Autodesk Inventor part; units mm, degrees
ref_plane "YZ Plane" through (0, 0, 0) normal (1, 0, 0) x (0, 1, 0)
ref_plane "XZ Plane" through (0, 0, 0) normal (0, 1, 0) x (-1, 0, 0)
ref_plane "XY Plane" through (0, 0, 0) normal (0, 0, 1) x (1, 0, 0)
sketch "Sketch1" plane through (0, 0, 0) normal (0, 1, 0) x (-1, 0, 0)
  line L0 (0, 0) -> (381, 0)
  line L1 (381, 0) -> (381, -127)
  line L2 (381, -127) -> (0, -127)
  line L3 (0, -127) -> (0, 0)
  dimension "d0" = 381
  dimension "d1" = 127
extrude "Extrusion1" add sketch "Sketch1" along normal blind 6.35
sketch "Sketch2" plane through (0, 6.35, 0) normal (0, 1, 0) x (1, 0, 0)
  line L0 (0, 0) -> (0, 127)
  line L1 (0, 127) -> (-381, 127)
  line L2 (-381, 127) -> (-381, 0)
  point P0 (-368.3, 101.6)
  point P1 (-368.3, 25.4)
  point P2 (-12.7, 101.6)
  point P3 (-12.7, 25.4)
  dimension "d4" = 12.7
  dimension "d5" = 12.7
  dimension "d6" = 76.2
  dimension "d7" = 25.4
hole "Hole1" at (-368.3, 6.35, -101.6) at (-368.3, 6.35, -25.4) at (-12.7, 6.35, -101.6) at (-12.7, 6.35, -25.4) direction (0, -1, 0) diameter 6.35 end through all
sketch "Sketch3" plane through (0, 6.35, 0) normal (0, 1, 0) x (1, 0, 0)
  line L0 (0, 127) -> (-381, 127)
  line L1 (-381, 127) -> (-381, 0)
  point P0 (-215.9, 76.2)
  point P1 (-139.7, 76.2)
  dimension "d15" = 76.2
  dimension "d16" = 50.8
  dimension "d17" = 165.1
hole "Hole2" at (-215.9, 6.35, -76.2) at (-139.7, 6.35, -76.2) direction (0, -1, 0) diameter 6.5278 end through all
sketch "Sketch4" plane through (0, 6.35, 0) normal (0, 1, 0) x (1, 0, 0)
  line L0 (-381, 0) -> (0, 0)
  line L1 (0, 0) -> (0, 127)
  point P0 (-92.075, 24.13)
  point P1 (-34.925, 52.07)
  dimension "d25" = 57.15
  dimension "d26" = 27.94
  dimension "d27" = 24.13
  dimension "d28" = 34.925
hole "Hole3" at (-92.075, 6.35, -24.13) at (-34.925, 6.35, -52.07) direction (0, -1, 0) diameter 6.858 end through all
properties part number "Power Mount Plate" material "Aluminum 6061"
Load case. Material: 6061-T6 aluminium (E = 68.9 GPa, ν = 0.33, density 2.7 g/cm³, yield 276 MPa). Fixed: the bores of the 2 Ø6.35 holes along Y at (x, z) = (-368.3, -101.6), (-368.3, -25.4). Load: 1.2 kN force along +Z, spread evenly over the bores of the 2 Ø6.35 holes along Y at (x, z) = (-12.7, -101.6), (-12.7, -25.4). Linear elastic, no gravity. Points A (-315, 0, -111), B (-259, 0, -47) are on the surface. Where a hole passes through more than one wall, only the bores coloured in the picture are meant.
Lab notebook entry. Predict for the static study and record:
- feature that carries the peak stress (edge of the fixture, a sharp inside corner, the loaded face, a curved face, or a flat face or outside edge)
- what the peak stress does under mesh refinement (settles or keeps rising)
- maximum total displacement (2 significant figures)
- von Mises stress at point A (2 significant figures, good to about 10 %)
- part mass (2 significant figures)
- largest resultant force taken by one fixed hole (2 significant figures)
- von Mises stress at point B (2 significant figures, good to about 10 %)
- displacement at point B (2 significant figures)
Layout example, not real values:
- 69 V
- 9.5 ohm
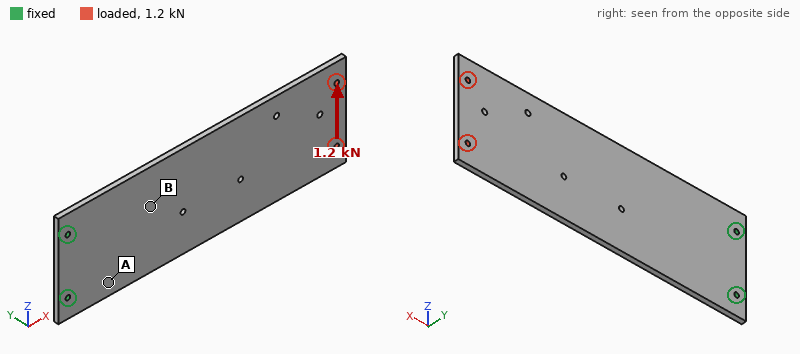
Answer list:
- edge of the fixture
- keeps rising
- 0.36 mm
- 16 MPa
- 830 g
- 5.4 kN
- 5.7 MPa
- 0.060 mm
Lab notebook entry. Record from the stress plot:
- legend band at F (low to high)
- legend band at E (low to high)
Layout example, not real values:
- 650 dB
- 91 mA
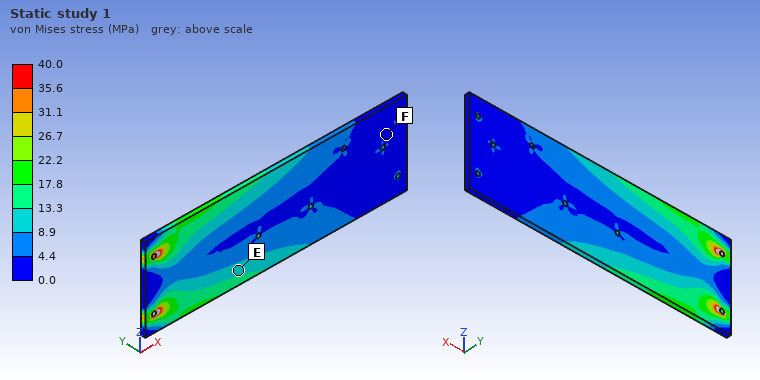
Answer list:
- 0.0 to 4.4 MPa
- 8.9 to 13.3 MPa
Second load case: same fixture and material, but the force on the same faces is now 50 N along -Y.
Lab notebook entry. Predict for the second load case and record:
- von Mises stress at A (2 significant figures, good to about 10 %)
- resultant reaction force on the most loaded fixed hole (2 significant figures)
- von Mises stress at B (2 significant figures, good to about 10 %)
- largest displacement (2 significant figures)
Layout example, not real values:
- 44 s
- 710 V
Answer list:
- 17 MPa
- 25 N
- 14 MPa
- 4.4 mm
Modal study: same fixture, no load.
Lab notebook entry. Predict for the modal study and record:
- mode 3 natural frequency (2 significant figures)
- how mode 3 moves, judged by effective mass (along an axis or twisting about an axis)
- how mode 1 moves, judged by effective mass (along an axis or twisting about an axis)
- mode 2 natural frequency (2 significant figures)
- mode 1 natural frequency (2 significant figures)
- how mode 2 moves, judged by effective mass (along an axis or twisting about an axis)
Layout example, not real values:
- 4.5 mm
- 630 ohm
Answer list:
- 230 Hz
- along Y
- along Y
- 220 Hz
- 37 Hz
- twisting about X
